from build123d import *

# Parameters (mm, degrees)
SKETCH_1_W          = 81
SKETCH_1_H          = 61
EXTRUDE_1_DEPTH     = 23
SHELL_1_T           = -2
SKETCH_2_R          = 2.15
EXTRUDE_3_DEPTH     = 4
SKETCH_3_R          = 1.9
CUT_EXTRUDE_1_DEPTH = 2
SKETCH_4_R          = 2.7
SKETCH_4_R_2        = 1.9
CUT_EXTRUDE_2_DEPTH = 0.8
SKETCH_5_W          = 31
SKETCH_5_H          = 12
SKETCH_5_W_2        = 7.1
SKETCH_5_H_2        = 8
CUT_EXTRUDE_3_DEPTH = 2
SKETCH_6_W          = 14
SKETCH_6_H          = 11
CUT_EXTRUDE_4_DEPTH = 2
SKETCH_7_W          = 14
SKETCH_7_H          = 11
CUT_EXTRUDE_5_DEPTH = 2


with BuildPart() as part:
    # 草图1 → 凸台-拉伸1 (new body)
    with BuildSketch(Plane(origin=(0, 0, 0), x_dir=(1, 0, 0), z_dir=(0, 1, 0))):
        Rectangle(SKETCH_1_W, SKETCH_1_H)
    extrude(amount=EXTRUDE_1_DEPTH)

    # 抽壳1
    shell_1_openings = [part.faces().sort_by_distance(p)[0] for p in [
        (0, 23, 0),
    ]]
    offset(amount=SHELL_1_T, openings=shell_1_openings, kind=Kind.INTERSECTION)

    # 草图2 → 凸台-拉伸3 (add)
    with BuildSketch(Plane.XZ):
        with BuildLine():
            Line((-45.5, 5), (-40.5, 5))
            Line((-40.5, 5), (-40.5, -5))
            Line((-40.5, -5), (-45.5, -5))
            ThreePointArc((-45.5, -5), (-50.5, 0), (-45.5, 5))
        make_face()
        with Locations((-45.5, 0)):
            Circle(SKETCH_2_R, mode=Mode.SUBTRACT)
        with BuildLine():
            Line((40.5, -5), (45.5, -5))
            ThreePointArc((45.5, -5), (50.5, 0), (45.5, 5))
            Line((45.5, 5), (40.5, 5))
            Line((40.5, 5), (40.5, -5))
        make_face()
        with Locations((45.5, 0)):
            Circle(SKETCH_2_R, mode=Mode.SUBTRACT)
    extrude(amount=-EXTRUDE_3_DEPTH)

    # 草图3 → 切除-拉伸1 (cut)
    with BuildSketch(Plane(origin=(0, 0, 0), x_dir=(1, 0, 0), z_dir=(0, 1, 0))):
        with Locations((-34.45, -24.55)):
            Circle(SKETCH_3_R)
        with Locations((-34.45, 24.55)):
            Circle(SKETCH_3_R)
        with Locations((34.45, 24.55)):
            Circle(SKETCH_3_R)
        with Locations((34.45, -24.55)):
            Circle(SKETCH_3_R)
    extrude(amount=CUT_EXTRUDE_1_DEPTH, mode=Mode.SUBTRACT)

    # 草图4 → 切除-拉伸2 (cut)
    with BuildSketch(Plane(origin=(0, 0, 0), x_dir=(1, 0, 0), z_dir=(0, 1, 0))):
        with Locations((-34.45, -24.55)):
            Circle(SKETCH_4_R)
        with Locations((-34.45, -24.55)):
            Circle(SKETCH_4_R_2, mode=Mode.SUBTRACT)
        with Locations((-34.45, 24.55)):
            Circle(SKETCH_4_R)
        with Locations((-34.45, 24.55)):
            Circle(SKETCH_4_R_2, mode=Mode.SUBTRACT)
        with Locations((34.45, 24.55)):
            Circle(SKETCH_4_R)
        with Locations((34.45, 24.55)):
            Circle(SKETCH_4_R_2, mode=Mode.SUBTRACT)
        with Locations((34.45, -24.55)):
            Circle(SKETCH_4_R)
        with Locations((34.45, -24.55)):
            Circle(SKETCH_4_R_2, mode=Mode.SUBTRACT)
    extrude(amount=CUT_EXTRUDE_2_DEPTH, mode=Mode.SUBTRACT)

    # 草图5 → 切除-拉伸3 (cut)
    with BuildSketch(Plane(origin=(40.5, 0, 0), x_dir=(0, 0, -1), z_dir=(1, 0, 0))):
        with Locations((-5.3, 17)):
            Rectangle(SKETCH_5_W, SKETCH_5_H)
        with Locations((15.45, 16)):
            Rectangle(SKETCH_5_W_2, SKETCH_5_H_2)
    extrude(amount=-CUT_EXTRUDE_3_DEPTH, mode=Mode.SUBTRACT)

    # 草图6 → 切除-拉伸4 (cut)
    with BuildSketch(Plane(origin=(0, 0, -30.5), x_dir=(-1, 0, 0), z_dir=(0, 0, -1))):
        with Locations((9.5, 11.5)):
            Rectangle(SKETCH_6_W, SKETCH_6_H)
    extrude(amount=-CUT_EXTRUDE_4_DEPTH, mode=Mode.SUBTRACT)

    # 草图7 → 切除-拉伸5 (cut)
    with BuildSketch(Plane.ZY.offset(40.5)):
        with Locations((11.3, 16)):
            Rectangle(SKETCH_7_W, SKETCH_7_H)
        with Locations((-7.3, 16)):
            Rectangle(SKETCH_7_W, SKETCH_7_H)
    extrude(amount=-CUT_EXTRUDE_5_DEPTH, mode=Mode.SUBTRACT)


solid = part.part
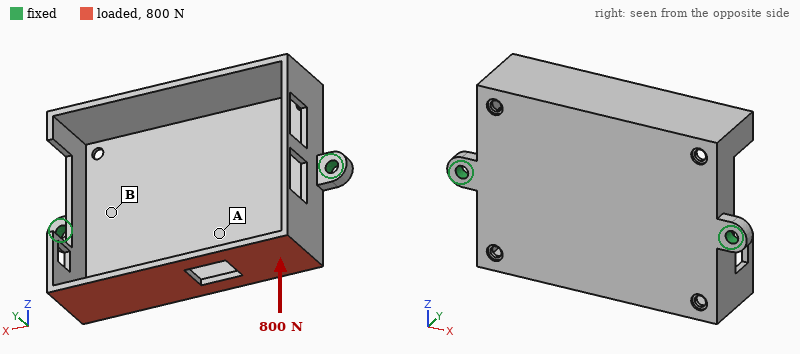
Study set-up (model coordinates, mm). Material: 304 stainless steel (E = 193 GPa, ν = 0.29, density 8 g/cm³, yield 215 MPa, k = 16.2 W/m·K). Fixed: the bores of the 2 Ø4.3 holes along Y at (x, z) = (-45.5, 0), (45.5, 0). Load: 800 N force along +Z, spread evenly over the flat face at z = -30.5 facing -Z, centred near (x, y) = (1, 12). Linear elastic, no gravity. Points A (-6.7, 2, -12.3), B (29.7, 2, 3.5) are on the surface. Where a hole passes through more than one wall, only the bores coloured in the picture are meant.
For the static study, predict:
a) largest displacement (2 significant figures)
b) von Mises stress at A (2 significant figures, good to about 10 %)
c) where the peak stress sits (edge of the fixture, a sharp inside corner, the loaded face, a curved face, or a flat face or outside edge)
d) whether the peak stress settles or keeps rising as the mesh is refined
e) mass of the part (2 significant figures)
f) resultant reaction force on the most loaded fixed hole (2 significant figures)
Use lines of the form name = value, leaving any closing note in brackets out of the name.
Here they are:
largest displacement = 0.19 mm
von Mises stress at A = 27 MPa
where the peak stress sits = edge of the fixture
whether the peak stress settles or keeps rising as the mesh is refined = keeps rising
mass of the part = 160 g
resultant reaction force on the most loaded fixed hole = 410 N
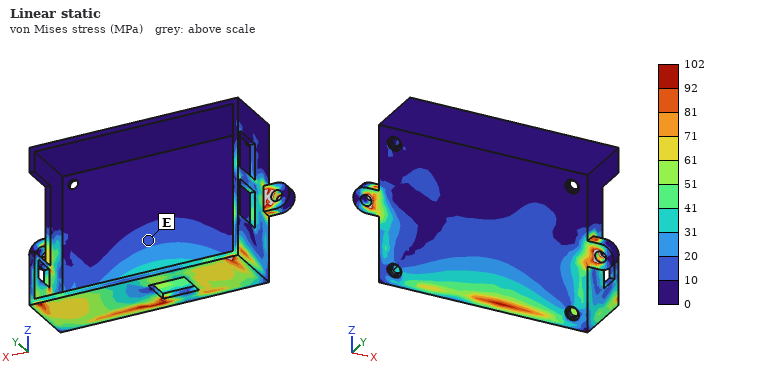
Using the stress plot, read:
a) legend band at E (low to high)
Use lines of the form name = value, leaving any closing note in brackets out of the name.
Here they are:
legend band at E = 10 to 20 MPa
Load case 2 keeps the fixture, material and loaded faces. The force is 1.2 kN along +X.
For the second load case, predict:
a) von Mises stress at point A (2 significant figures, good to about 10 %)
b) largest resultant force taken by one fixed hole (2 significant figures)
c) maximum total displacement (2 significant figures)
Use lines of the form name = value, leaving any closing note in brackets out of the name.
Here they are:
von Mises stress at point A = 21 MPa
largest resultant force taken by one fixed hole = 760 N
maximum total displacement = 82 µm
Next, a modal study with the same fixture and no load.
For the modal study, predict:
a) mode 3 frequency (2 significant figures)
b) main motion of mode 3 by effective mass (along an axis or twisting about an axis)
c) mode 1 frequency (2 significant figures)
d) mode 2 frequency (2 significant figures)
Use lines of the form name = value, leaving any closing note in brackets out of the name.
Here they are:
mode 3 frequency = 2300 Hz
main motion of mode 3 by effective mass = along Y
mode 1 frequency = 1200 Hz
mode 2 frequency = 1900 Hz
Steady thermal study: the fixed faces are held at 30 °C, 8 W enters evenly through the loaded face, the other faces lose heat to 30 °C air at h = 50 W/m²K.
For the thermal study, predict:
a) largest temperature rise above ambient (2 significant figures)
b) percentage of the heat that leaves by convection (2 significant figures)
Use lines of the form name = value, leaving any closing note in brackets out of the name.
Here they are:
largest temperature rise above ambient = 41 K
percentage of the heat that leaves by convection = 94 %
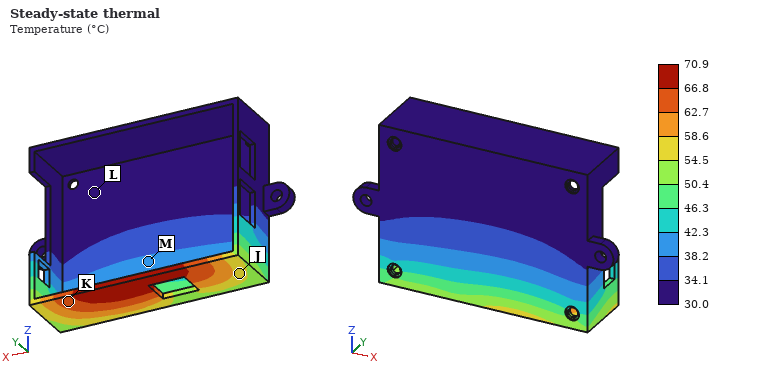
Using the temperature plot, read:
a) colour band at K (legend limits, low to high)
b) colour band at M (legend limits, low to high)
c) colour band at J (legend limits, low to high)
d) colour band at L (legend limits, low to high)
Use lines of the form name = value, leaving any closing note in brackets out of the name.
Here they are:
colour band at K = 62.7 to 66.8 °C
colour band at M = 38.2 to 42.3 °C
colour band at J = 54.5 to 58.6 °C
colour band at L = 30.0 to 34.1 °C
